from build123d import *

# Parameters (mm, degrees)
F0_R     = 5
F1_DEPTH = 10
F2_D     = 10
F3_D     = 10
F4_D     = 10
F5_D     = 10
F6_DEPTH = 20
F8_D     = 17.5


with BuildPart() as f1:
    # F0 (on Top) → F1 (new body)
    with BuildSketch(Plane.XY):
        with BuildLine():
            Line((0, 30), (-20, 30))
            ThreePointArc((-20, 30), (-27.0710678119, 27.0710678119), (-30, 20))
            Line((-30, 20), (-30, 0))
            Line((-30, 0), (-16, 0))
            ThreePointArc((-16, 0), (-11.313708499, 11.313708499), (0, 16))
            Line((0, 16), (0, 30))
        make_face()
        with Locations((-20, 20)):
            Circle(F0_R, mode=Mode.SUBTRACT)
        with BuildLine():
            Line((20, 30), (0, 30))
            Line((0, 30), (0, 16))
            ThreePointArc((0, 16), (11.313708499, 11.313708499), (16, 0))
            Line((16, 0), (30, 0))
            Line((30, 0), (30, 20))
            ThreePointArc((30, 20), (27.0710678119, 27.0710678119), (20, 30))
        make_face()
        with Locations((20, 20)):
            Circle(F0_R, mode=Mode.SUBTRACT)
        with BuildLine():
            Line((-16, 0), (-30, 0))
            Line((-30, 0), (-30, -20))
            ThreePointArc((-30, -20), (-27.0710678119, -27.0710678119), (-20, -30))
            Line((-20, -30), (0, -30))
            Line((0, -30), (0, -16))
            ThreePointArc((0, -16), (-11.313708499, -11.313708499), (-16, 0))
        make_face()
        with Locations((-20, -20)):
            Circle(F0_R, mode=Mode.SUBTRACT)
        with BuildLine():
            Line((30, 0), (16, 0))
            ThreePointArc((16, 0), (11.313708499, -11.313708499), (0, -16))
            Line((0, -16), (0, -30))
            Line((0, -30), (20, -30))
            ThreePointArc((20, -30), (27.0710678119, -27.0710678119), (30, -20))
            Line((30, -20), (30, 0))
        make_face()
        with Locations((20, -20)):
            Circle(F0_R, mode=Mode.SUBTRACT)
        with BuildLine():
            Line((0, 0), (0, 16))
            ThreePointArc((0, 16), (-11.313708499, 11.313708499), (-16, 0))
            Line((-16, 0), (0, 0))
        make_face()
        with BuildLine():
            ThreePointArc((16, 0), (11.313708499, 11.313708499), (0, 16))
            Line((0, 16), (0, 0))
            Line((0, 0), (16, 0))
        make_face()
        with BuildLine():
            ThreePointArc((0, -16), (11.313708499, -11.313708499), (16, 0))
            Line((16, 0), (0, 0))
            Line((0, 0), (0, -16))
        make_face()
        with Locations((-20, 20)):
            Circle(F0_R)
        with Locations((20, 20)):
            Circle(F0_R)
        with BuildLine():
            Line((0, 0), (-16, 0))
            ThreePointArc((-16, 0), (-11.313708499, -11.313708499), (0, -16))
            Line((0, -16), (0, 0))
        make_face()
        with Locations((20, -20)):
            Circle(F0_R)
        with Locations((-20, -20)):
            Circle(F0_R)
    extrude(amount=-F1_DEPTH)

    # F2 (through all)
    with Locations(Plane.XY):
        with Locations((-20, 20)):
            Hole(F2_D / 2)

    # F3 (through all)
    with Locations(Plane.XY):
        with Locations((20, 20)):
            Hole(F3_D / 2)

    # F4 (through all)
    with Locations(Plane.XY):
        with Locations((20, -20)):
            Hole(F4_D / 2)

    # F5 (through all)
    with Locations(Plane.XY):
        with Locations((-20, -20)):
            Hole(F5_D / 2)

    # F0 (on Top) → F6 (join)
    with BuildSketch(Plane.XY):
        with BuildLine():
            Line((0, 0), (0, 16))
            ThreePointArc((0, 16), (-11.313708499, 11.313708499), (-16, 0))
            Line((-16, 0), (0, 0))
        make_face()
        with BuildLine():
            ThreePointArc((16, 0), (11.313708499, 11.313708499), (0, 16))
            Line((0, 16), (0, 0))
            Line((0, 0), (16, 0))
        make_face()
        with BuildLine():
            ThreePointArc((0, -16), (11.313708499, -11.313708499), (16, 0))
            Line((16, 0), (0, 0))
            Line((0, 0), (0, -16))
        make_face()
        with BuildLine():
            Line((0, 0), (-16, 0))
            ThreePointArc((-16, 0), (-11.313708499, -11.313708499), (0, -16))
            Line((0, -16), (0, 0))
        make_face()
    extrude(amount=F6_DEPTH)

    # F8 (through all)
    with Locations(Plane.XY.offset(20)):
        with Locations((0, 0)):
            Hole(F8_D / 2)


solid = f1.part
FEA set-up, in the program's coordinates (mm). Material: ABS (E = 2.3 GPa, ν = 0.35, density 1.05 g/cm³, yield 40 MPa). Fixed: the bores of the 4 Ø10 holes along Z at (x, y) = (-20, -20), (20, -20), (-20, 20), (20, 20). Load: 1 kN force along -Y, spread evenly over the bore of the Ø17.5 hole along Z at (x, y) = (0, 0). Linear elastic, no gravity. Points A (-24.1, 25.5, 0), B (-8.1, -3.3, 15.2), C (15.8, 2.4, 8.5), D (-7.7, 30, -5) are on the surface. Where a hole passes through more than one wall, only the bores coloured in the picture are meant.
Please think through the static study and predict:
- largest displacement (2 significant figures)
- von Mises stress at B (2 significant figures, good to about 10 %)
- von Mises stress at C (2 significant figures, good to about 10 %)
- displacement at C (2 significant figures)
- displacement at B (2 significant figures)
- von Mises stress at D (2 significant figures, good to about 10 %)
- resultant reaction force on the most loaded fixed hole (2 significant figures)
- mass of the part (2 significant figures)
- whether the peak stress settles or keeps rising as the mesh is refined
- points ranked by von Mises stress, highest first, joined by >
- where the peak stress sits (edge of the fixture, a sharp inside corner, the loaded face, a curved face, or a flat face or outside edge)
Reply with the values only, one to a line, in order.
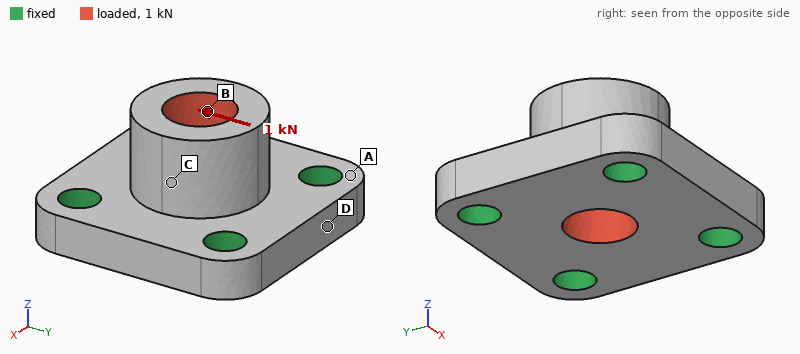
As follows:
73 µm
2.1 MPa
1.4 MPa
37 µm
56 µm
0.84 MPa
310 N
43 g
keeps rising
B > C > D > A
edge of the fixture
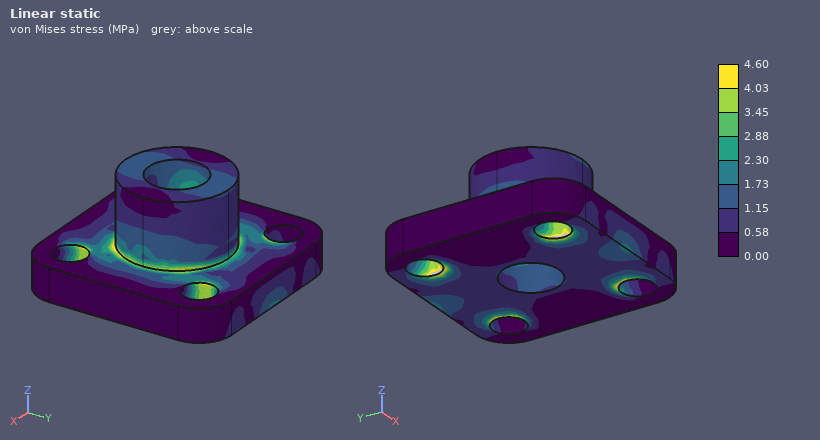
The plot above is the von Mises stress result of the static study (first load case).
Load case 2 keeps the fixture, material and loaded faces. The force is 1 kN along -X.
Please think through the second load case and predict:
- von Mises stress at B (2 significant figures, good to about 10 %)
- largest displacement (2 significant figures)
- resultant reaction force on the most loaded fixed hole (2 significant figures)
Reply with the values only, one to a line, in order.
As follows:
1.1 MPa
73 µm
310 N
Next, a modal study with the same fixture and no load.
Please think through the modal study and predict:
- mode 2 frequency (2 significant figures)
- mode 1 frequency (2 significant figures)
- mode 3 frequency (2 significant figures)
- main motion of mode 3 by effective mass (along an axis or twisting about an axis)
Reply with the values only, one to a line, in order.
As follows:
5100 Hz
5000 Hz
5900 Hz
along Z
